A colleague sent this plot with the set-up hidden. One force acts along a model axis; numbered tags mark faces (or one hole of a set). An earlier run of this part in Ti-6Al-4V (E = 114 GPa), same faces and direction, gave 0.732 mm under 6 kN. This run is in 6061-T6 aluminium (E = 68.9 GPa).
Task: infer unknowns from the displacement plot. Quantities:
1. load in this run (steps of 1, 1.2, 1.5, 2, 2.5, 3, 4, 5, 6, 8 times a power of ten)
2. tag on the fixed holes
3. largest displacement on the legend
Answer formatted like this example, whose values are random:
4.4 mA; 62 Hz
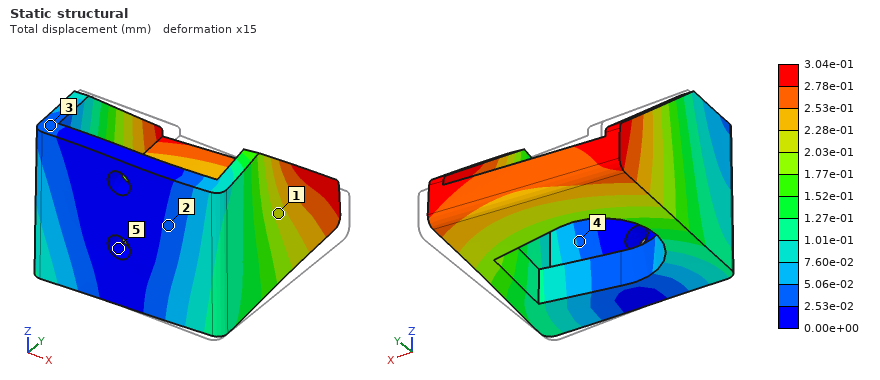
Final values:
1.5 kN; 5; 3.04e-01 mm
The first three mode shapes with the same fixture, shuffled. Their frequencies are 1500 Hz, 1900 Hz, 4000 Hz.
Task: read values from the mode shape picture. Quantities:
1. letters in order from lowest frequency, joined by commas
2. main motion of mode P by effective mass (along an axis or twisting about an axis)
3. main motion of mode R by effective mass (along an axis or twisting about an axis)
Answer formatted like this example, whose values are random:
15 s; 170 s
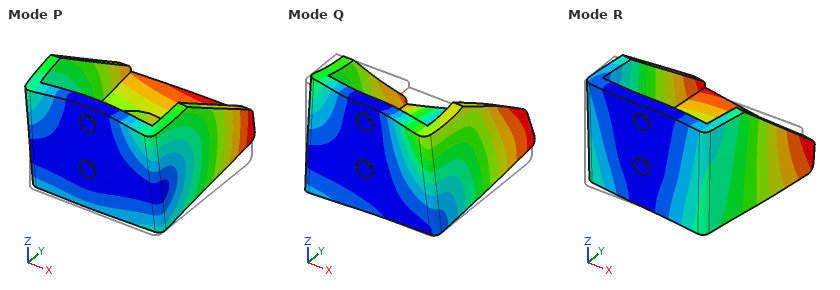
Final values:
R, P, Q; along Z; along X
